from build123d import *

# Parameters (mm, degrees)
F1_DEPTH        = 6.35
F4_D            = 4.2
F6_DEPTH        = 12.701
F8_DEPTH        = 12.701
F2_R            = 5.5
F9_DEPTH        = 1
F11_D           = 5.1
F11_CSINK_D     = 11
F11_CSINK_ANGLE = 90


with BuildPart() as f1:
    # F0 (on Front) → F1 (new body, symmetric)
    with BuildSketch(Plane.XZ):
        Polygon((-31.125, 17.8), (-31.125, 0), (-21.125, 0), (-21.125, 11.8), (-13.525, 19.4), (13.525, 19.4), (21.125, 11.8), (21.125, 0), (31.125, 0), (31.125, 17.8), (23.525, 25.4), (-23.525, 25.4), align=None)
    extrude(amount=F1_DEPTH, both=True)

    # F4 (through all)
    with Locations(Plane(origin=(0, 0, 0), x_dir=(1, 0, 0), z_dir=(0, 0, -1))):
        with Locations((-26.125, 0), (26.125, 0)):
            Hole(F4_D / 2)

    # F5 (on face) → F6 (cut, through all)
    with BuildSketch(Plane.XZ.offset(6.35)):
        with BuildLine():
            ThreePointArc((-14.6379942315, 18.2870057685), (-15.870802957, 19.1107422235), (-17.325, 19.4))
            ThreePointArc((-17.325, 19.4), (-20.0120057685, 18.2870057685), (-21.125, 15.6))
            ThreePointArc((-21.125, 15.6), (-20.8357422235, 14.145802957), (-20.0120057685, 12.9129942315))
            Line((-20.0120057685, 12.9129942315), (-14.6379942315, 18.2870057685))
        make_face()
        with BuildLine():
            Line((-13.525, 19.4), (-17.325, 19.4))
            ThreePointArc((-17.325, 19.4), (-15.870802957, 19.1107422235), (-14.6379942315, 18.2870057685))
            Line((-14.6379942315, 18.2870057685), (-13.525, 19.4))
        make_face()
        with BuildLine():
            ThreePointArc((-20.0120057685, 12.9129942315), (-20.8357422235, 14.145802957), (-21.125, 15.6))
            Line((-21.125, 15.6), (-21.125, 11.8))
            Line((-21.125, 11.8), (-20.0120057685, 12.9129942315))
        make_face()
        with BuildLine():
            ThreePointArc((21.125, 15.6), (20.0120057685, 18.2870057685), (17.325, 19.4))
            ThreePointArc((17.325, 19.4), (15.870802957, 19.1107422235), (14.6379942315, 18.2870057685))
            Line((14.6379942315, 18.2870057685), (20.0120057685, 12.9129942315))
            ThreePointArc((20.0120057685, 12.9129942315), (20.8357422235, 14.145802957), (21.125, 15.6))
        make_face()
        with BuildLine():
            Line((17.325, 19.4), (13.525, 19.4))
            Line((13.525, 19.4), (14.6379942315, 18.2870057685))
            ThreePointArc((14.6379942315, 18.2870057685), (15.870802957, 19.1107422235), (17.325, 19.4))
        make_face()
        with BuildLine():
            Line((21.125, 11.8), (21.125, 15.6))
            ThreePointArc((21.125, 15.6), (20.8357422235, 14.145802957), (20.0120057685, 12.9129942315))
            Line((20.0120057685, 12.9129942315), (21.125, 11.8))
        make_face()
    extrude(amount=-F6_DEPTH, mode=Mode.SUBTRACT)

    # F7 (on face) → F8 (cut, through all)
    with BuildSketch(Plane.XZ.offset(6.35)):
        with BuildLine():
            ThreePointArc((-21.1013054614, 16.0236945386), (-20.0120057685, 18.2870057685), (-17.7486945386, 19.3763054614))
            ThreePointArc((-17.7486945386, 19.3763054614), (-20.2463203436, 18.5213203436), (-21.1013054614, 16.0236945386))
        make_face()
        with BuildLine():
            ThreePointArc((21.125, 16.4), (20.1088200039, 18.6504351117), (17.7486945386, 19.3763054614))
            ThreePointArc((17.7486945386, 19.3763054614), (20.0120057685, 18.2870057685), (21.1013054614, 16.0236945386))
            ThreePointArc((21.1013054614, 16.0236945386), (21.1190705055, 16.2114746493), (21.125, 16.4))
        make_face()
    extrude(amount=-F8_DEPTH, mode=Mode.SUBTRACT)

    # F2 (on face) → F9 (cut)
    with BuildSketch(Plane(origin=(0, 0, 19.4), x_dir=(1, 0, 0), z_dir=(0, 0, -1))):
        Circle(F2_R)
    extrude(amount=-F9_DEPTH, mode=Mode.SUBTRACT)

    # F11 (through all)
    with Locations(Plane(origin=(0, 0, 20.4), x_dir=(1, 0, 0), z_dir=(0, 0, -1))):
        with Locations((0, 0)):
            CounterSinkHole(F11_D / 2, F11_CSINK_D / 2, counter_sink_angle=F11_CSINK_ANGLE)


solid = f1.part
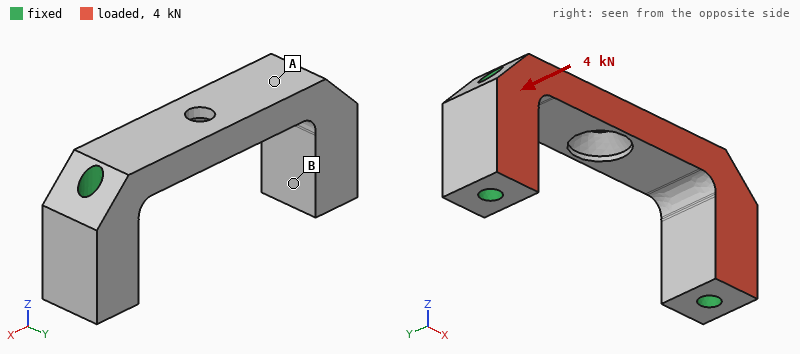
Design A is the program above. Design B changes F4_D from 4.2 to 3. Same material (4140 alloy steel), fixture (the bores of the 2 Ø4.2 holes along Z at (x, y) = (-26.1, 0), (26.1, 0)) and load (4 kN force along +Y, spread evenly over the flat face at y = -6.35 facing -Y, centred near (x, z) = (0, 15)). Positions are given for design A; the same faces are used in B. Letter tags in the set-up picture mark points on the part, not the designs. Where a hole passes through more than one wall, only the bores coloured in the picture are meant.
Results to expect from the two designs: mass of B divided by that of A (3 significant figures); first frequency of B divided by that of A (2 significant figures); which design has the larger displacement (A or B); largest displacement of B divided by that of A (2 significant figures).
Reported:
1.04
0.97
B
1.2
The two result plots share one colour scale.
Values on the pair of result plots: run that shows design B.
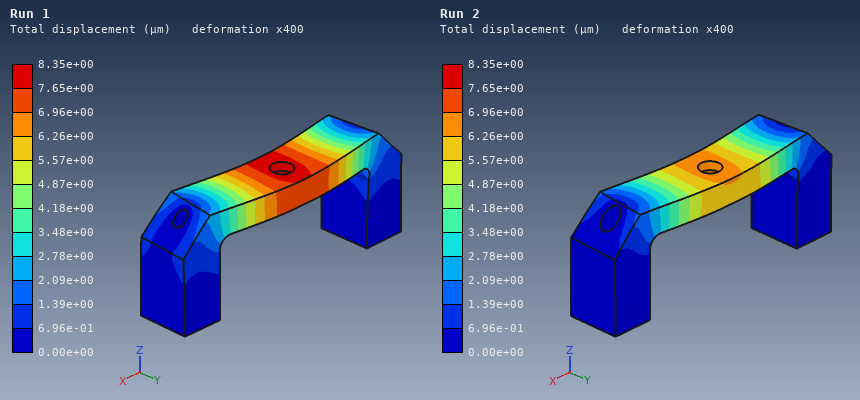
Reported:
Run 1
